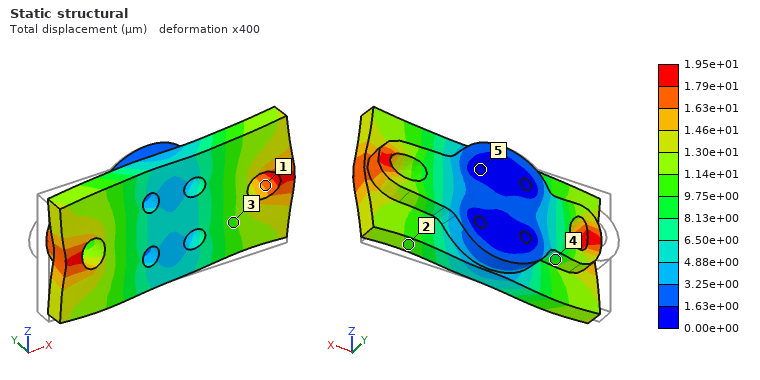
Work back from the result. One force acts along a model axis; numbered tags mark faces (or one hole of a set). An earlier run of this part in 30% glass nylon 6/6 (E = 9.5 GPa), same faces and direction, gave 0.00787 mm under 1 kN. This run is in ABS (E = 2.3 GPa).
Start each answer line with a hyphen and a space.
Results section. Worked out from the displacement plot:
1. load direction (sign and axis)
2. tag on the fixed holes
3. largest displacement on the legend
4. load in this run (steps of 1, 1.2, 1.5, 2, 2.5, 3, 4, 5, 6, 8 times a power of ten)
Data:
- +X
- 5
- 1.95e+01 µm
- 600 N
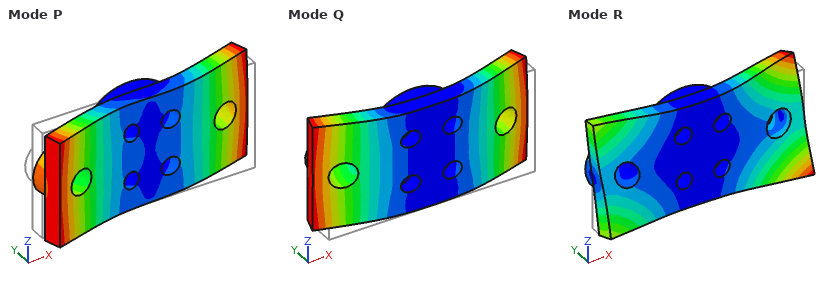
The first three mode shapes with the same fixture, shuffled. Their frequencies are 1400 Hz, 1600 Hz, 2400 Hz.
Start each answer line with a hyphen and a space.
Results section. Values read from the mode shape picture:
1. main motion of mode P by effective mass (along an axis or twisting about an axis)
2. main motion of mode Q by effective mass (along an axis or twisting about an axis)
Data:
- twisting about Z
- along Y
